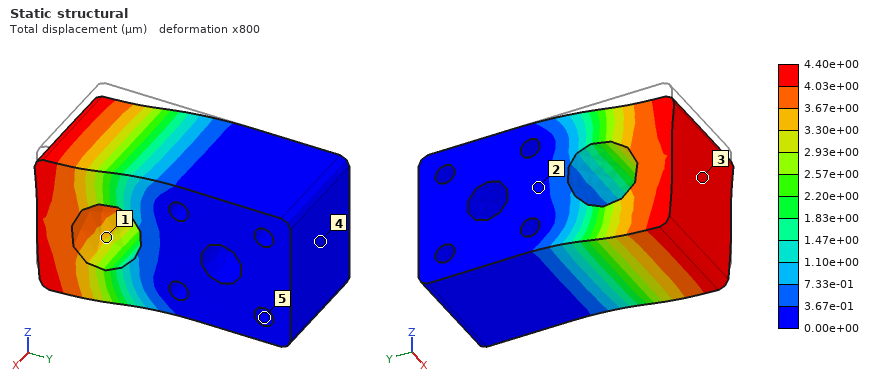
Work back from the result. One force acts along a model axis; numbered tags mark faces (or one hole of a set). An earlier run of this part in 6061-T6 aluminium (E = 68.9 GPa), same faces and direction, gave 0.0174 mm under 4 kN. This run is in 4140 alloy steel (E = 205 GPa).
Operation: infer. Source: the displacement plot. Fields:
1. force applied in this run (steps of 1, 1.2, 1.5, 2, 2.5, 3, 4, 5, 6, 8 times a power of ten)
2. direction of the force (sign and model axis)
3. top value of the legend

3 kN
-Z
4.40e+00 µm
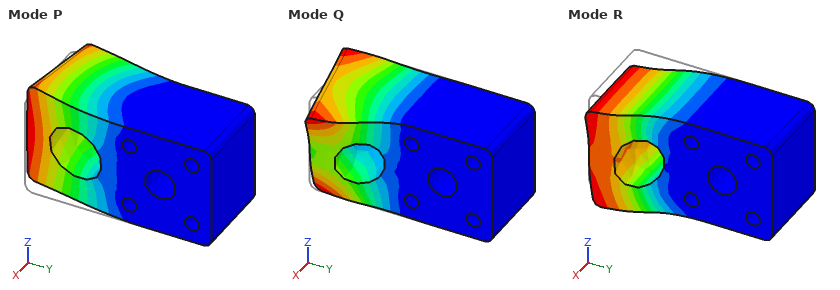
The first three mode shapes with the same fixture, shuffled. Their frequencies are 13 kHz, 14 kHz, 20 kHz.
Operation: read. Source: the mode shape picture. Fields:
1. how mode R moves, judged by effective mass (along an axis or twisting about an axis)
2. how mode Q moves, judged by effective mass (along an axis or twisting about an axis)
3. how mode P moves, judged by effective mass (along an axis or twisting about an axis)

along Z
twisting about Y
along X
